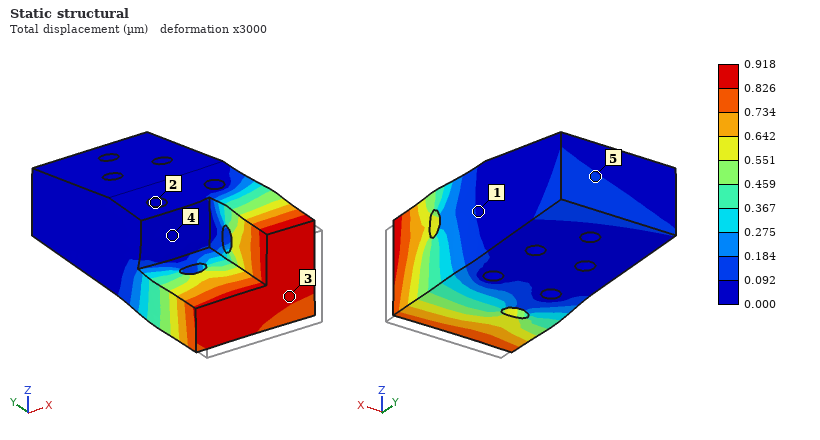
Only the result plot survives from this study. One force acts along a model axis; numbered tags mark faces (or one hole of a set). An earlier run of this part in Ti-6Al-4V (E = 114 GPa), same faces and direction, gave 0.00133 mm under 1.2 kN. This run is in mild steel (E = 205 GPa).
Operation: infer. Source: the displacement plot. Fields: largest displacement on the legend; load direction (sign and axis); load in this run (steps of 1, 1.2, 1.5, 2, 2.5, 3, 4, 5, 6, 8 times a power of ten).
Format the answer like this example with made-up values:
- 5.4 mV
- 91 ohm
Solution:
- 0.918 µm
- +Y
- 1.5 kN
